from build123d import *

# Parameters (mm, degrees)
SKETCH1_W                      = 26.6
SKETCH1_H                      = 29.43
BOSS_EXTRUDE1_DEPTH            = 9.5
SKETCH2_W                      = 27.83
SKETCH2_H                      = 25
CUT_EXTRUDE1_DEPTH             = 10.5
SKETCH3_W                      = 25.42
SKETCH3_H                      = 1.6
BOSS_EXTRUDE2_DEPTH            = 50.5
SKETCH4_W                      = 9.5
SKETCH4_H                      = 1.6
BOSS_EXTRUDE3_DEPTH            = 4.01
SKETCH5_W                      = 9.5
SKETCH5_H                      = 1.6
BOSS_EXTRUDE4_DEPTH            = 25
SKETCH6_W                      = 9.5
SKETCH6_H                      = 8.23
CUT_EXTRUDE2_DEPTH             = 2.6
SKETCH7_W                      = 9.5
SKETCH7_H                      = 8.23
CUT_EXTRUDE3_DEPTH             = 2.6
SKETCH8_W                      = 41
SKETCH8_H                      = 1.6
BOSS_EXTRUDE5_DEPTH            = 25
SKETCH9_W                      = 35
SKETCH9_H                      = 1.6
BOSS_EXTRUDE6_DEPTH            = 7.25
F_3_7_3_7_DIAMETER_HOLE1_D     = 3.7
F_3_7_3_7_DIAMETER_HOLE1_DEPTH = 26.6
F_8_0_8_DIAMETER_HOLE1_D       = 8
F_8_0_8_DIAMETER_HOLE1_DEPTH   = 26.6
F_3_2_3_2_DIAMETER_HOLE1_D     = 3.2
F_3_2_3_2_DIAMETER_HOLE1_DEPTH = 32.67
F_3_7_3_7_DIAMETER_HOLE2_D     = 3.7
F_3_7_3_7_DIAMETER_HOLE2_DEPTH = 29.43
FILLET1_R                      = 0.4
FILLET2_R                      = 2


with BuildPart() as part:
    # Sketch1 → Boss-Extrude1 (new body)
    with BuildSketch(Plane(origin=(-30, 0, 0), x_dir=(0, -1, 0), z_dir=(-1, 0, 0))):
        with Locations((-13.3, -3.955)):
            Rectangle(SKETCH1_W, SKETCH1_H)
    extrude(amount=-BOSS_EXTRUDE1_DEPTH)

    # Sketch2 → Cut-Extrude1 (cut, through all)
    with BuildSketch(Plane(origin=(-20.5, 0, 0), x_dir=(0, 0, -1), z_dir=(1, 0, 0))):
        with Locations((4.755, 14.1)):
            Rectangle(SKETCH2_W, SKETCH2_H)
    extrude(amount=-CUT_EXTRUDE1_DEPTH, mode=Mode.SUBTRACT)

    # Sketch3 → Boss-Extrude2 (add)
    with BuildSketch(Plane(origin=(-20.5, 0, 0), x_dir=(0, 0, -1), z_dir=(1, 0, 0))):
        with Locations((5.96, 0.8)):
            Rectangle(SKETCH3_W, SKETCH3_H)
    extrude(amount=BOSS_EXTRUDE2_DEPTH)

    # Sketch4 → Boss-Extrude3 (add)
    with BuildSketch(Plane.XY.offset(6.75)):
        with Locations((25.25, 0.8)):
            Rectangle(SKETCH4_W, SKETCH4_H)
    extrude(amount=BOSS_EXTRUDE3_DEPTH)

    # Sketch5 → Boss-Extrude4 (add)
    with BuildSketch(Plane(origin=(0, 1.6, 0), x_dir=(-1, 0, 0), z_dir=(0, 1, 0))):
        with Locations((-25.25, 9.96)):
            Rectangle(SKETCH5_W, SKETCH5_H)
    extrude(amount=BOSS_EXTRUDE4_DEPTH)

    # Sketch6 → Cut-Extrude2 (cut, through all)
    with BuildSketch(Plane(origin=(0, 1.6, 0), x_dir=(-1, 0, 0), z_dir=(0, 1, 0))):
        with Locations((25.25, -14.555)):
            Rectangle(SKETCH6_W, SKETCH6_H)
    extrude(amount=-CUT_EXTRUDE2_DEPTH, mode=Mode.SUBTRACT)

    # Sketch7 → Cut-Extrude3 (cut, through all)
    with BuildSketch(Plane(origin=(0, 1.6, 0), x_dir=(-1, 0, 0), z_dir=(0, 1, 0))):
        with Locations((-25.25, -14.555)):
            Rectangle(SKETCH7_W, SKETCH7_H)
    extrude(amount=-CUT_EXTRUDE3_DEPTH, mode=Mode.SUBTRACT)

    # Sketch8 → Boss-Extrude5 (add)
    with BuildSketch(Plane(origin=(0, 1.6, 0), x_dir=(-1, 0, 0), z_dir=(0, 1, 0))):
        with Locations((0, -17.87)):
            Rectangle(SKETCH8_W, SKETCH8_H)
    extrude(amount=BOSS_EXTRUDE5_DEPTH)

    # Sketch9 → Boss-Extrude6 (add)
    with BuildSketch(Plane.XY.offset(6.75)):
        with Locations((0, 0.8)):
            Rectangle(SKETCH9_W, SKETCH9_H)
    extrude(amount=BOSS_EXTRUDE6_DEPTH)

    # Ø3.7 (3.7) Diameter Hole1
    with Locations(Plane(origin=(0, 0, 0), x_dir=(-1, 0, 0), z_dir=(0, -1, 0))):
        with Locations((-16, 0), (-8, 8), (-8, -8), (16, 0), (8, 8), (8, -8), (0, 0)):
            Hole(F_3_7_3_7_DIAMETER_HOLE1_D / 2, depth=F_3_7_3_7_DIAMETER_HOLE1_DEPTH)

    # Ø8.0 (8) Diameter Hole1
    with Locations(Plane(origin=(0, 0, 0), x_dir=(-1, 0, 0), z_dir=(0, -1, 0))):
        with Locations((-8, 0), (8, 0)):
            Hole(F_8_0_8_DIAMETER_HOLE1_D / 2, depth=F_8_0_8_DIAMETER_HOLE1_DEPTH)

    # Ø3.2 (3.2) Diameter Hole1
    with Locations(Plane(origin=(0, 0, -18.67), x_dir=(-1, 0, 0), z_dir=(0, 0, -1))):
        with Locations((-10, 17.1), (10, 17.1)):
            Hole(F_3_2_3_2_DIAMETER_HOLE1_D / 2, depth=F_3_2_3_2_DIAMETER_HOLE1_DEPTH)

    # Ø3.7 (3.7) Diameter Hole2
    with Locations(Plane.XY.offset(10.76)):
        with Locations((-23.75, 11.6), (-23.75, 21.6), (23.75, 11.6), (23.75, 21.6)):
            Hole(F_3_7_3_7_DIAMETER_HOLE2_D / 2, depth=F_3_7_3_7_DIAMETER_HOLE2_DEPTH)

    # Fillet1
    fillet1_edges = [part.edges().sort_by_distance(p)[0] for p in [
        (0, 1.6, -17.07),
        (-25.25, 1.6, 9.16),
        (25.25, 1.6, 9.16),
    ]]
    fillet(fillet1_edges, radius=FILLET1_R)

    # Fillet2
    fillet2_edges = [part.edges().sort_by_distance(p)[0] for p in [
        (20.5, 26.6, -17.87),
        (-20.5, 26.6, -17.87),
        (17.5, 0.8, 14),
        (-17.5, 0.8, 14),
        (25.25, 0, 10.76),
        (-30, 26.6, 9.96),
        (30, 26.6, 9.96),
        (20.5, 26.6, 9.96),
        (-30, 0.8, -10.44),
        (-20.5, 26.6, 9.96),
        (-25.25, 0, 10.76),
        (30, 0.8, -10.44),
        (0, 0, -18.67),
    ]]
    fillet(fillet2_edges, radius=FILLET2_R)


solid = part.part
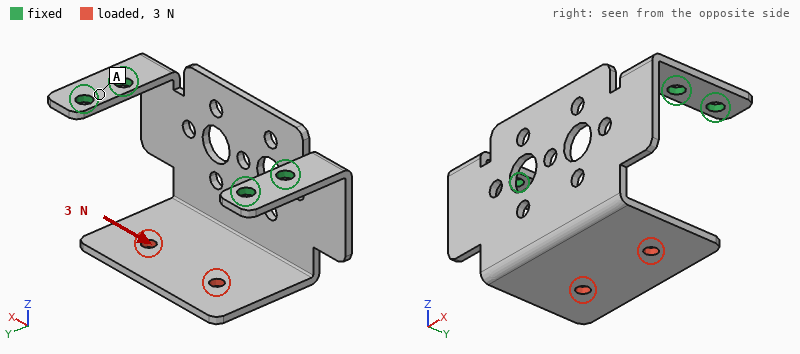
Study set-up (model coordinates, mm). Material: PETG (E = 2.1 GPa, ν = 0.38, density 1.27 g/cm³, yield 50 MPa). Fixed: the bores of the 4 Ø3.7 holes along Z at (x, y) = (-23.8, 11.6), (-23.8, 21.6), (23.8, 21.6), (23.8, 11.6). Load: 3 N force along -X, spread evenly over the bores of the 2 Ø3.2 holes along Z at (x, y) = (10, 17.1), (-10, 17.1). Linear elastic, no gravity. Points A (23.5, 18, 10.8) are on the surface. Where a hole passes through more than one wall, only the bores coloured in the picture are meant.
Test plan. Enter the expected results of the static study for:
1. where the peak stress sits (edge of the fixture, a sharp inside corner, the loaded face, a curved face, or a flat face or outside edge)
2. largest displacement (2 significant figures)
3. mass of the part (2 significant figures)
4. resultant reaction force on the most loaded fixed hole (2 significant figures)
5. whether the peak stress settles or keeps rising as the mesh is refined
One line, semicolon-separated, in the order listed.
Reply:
edge of the fixture; 0.80 mm; 5.9 g; 2.9 N; keeps rising
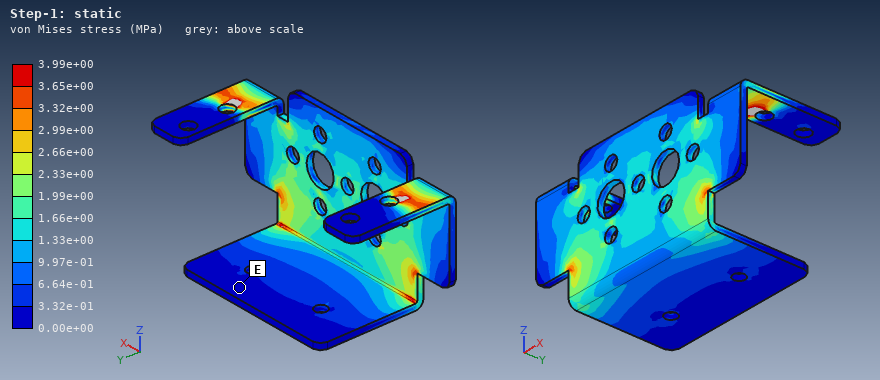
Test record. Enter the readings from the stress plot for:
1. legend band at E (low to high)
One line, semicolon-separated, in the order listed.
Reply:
0.00e+00 to 3.32e-01 MPa
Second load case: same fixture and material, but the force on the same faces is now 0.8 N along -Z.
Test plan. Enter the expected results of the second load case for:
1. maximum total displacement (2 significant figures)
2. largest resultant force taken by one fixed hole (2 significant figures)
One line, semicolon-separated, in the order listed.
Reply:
0.75 mm; 0.41 N
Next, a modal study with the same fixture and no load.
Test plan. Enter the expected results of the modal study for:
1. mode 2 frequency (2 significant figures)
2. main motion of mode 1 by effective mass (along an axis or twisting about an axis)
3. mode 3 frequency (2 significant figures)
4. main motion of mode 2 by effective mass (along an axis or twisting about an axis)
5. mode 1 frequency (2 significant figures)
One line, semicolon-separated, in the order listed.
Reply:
240 Hz; along Y; 300 Hz; along X; 89 Hz
